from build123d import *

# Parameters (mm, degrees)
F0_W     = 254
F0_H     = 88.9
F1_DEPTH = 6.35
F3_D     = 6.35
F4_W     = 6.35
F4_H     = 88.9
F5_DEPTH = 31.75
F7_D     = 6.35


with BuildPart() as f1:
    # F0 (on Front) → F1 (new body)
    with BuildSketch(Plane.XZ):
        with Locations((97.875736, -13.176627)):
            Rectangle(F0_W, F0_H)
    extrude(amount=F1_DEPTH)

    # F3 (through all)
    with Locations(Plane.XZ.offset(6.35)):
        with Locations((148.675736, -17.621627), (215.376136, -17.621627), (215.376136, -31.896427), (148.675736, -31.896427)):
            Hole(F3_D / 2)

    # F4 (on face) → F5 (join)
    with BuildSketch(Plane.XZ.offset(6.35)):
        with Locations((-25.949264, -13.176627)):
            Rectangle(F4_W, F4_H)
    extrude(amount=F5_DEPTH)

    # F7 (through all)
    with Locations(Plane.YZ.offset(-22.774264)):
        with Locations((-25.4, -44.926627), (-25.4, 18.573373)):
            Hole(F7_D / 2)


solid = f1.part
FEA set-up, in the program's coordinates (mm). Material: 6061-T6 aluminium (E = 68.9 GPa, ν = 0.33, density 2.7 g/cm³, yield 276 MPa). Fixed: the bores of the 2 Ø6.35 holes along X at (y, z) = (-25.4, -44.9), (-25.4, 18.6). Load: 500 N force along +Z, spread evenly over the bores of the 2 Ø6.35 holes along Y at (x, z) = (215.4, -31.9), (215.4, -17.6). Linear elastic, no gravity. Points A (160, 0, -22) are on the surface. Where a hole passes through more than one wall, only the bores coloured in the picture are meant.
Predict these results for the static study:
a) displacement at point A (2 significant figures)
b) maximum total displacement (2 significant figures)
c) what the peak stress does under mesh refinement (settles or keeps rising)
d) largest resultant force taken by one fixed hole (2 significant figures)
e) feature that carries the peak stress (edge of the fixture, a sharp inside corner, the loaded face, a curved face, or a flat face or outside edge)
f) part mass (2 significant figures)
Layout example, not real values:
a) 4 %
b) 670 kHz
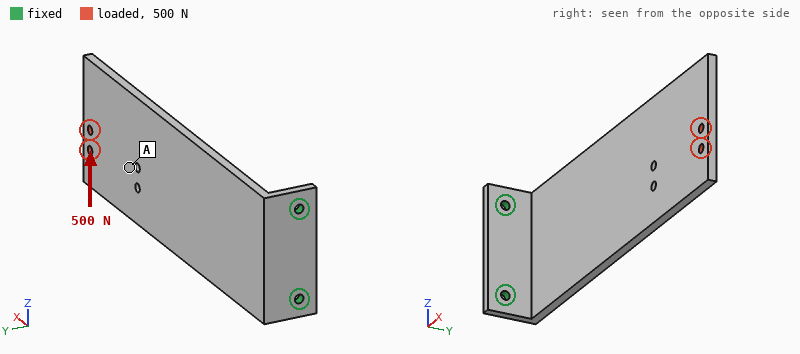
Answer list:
a) 0.53 mm
b) 0.77 mm
c) keeps rising
d) 1.8 kN
e) edge of the fixture
f) 430 g
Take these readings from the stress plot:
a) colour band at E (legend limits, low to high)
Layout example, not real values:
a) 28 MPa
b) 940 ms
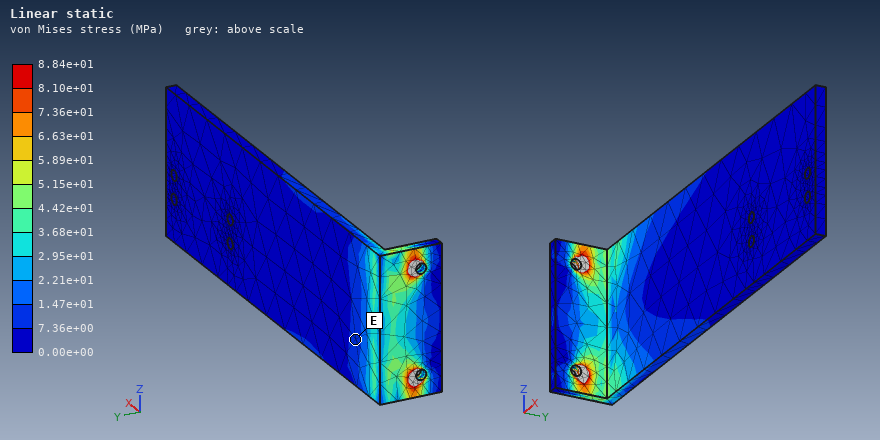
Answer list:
a) 7.36e+00 to 1.47e+01 MPa
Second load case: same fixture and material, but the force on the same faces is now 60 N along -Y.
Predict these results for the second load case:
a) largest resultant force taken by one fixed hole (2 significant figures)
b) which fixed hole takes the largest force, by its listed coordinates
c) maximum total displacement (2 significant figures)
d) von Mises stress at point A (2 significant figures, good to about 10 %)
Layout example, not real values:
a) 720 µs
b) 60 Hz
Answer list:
a) 78 N
b) (-25.4, -44.9)
c) 2.8 mm
d) 5.6 MPa
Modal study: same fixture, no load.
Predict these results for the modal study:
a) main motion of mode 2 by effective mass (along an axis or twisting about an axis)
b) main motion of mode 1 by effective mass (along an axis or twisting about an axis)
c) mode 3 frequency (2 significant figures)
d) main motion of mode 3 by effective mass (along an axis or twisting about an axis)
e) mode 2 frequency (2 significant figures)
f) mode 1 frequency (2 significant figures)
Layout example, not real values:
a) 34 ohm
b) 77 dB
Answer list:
a) along Z
b) along Y
c) 460 Hz
d) along Y
e) 350 Hz
f) 73 Hz
